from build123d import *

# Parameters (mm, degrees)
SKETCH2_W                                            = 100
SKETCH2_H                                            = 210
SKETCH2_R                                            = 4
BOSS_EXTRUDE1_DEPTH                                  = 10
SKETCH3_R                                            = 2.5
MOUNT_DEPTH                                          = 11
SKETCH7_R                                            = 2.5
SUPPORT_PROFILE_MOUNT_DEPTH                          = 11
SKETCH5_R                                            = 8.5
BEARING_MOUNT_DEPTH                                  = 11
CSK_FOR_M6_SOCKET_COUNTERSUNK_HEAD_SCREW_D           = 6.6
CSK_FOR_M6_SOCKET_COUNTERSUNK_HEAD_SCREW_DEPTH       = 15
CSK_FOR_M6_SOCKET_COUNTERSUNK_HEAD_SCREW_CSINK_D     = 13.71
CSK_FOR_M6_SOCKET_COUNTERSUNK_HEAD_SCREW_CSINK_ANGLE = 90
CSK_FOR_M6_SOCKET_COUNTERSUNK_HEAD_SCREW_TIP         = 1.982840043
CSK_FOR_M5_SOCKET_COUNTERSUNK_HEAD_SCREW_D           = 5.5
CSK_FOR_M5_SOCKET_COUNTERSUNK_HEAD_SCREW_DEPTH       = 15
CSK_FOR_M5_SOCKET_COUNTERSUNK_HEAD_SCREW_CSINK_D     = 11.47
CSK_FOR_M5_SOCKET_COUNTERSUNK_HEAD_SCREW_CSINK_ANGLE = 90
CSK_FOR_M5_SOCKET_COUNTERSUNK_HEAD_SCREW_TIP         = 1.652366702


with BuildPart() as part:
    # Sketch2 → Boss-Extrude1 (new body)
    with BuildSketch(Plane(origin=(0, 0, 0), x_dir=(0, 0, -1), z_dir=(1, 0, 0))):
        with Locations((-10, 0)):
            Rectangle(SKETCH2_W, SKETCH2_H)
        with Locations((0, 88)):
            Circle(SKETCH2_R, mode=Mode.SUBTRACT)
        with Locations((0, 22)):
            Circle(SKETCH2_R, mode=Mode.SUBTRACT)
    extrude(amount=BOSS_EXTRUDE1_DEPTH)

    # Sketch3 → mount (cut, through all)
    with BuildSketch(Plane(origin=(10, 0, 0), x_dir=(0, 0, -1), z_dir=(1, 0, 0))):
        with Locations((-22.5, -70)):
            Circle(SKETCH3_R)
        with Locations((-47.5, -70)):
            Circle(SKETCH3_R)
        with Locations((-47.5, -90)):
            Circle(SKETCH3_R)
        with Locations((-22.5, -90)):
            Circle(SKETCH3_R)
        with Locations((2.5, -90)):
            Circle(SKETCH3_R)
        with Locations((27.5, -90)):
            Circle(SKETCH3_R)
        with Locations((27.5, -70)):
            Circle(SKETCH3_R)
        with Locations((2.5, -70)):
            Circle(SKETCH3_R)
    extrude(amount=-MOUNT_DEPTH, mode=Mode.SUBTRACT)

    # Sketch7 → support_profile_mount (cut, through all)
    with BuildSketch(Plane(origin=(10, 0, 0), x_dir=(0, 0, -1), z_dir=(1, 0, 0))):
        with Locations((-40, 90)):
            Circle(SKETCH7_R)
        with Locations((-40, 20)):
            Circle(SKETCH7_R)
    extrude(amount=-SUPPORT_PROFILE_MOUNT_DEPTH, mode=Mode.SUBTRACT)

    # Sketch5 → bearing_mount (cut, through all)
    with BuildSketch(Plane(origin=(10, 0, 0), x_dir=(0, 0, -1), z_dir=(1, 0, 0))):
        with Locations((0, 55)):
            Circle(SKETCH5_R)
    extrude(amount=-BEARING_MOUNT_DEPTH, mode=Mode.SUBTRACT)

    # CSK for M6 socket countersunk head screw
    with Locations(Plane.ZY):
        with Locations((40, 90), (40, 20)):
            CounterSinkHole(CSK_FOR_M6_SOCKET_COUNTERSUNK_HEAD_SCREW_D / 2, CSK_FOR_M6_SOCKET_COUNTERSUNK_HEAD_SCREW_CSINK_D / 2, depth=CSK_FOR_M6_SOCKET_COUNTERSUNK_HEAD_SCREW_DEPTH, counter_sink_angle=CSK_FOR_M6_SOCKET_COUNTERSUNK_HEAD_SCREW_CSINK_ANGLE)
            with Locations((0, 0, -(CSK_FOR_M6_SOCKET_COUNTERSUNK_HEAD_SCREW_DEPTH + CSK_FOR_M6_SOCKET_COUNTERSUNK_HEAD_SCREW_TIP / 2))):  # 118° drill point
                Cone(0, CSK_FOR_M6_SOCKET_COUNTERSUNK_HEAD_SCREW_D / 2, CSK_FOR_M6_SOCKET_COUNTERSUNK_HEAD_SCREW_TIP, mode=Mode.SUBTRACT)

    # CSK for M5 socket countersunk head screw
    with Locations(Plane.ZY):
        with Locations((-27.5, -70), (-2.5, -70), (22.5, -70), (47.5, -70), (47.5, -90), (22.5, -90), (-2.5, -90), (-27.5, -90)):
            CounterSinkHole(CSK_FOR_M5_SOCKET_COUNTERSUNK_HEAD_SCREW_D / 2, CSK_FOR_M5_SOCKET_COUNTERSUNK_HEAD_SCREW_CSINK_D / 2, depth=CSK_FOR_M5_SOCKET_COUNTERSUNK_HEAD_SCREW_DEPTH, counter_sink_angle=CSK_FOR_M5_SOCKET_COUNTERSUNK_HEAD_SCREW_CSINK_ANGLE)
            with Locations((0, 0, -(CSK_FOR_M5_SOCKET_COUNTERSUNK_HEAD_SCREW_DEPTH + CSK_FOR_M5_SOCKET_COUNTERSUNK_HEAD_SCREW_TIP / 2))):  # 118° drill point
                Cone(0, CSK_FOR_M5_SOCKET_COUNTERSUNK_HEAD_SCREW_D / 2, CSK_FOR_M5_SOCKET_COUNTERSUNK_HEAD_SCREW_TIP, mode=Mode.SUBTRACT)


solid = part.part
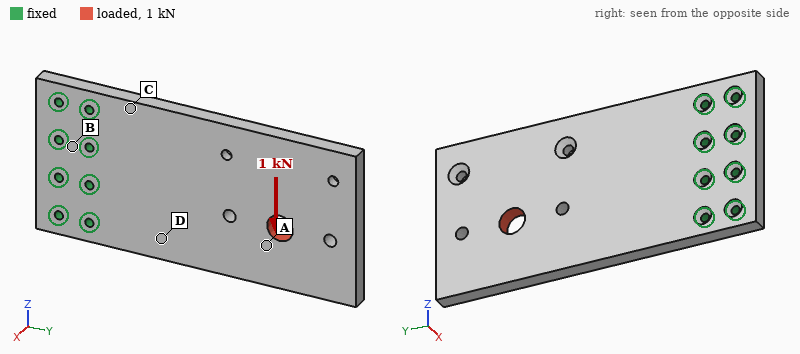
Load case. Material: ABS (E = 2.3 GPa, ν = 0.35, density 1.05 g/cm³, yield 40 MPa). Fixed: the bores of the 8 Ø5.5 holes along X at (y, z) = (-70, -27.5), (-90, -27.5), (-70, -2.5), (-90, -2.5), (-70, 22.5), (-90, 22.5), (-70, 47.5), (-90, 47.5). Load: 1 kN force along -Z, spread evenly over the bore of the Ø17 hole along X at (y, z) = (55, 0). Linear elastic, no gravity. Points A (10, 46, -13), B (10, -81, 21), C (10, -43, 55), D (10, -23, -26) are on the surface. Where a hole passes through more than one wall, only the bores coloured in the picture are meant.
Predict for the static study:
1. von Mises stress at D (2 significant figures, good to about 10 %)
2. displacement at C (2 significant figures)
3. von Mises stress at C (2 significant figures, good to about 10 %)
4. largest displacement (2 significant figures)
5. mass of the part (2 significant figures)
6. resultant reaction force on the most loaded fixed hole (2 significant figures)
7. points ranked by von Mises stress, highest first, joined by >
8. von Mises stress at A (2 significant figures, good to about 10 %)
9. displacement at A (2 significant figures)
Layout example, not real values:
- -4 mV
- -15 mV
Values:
- 3.7 MPa
- 0.13 mm
- 5.5 MPa
- 0.84 mm
- 210 g
- 1.2 kN
- C > D > A > B
- 2.3 MPa
- 0.53 mm
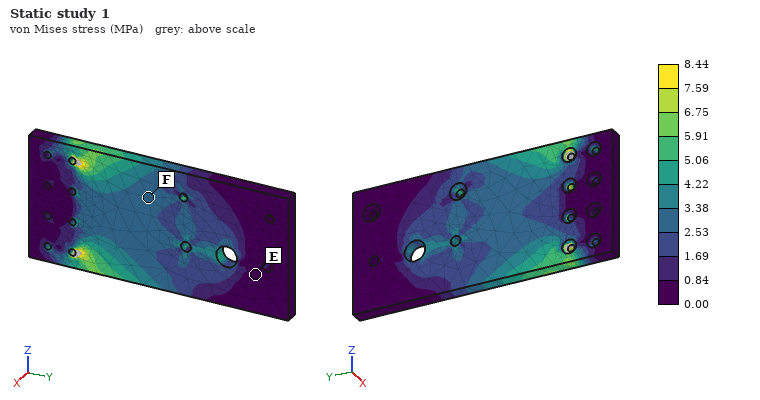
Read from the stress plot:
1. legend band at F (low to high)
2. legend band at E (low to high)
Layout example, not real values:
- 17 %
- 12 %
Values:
- 2.53 to 3.38 MPa
- 0.00 to 0.84 MPa
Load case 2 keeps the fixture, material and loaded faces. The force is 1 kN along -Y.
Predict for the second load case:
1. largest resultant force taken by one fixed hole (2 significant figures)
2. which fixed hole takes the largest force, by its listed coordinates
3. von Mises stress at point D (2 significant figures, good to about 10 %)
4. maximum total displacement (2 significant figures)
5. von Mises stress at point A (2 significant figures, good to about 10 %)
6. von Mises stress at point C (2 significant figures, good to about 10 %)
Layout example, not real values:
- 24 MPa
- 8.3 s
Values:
- 310 N
- (-70, -27.5)
- 1.4 MPa
- 0.13 mm
- 1.8 MPa
- 0.38 MPa
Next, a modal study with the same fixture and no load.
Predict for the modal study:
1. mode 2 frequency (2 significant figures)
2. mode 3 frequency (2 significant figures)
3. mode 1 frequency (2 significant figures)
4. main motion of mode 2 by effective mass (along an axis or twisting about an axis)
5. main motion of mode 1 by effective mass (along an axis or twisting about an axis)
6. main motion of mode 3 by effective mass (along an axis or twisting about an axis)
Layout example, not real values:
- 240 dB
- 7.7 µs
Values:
- 280 Hz
- 470 Hz
- 78 Hz
- twisting about Y
- along X
- along X
